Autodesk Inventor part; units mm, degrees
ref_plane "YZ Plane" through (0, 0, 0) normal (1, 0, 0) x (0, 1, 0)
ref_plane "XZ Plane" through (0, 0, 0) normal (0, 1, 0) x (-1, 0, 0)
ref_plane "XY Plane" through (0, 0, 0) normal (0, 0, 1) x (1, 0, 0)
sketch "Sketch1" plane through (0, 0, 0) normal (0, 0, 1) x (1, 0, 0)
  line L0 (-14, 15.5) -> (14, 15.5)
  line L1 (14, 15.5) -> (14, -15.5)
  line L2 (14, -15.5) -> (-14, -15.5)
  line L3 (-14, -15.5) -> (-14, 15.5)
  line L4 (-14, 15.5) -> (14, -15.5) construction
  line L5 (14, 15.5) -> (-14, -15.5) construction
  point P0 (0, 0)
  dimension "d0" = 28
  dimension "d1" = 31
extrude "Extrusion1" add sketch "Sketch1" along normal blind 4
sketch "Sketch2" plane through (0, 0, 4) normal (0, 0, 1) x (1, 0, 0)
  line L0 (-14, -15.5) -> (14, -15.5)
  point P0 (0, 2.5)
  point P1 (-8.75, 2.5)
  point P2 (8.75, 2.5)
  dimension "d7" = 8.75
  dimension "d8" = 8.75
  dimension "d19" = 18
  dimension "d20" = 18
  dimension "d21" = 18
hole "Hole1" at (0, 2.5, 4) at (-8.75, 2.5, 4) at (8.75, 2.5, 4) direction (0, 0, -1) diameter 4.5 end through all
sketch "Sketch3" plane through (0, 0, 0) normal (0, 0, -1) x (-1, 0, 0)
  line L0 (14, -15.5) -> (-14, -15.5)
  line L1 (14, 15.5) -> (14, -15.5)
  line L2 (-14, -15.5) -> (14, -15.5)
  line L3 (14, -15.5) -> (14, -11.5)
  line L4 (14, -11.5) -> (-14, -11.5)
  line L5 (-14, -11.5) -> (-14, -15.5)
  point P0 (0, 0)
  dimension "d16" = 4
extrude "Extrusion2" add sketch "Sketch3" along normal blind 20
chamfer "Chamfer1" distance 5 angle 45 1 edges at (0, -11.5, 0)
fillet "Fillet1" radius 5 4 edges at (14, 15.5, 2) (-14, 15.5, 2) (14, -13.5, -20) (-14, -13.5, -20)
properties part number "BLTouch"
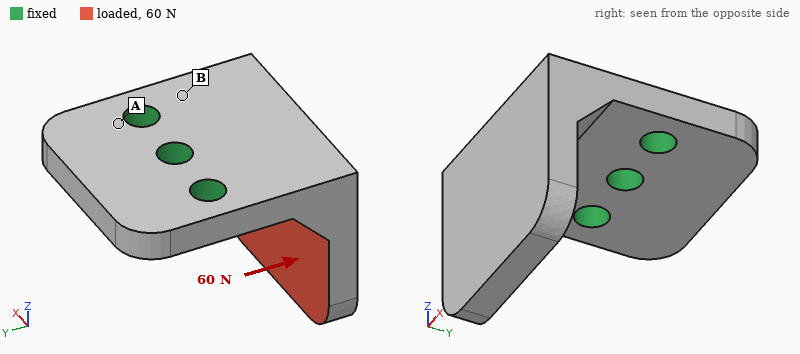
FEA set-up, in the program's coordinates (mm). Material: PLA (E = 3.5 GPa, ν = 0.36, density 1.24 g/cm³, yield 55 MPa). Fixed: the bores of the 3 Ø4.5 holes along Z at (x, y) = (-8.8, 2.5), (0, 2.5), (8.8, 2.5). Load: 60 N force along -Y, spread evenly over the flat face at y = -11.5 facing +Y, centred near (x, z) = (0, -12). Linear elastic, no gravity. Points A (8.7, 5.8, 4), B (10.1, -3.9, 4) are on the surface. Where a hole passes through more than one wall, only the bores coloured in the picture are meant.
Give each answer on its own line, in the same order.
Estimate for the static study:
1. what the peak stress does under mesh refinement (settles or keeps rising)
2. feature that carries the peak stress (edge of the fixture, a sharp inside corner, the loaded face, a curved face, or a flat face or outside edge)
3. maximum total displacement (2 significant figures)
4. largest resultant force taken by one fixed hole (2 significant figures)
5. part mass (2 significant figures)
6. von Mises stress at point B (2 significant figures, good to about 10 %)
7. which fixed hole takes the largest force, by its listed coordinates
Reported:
keeps rising
edge of the fixture
0.46 mm
24 N
7.2 g
10.0 MPa
(0, 2.5)
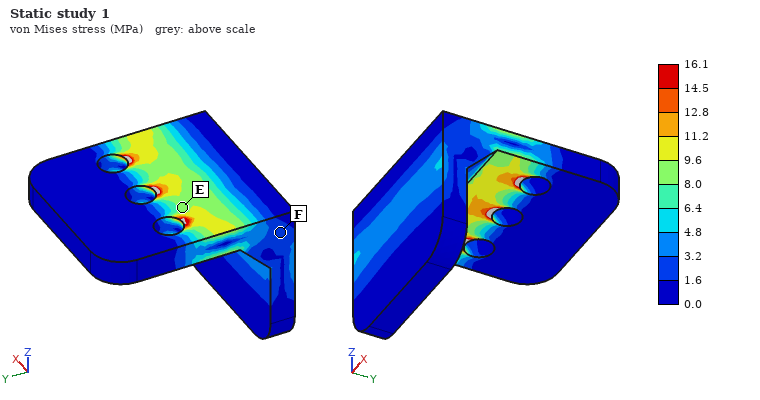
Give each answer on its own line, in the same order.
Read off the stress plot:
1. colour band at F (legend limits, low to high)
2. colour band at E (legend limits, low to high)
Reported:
1.6 to 3.2 MPa
8.0 to 9.6 MPa
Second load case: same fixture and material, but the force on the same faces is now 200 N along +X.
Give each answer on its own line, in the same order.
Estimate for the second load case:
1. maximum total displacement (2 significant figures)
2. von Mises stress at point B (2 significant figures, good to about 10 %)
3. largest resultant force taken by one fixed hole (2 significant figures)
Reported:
0.43 mm
11 MPa
200 N
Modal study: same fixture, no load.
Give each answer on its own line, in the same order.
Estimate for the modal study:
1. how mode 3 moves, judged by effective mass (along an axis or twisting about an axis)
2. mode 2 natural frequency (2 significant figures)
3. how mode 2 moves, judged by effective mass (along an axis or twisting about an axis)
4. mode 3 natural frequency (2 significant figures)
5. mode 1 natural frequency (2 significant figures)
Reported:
along Z
2500 Hz
along X
4300 Hz
1300 Hz
